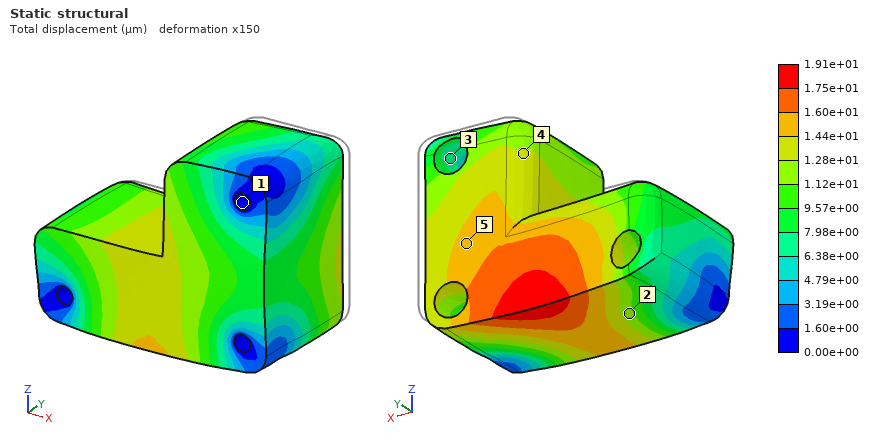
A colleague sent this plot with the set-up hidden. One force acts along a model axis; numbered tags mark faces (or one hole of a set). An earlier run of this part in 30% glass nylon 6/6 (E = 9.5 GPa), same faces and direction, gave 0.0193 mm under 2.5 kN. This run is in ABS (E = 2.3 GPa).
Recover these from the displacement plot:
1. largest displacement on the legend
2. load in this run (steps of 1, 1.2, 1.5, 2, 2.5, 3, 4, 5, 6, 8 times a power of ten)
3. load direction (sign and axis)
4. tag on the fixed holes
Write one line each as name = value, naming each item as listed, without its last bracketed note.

largest displacement on the legend = 1.91e+01 µm
load in this run = 600 N
load direction = -Y
tag on the fixed holes = 1
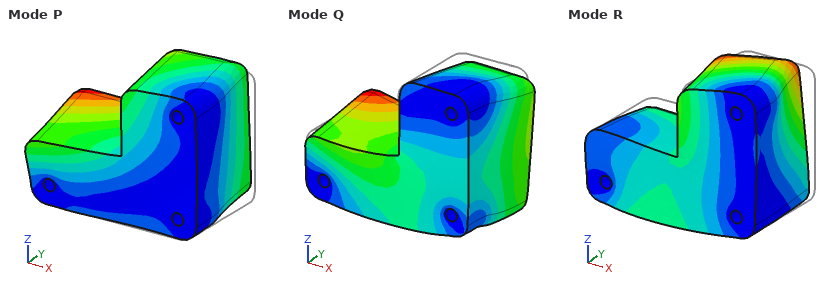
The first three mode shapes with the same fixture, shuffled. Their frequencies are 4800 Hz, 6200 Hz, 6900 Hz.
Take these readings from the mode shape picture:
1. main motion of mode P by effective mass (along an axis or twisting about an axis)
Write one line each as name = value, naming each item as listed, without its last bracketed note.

main motion of mode P by effective mass = along Z
